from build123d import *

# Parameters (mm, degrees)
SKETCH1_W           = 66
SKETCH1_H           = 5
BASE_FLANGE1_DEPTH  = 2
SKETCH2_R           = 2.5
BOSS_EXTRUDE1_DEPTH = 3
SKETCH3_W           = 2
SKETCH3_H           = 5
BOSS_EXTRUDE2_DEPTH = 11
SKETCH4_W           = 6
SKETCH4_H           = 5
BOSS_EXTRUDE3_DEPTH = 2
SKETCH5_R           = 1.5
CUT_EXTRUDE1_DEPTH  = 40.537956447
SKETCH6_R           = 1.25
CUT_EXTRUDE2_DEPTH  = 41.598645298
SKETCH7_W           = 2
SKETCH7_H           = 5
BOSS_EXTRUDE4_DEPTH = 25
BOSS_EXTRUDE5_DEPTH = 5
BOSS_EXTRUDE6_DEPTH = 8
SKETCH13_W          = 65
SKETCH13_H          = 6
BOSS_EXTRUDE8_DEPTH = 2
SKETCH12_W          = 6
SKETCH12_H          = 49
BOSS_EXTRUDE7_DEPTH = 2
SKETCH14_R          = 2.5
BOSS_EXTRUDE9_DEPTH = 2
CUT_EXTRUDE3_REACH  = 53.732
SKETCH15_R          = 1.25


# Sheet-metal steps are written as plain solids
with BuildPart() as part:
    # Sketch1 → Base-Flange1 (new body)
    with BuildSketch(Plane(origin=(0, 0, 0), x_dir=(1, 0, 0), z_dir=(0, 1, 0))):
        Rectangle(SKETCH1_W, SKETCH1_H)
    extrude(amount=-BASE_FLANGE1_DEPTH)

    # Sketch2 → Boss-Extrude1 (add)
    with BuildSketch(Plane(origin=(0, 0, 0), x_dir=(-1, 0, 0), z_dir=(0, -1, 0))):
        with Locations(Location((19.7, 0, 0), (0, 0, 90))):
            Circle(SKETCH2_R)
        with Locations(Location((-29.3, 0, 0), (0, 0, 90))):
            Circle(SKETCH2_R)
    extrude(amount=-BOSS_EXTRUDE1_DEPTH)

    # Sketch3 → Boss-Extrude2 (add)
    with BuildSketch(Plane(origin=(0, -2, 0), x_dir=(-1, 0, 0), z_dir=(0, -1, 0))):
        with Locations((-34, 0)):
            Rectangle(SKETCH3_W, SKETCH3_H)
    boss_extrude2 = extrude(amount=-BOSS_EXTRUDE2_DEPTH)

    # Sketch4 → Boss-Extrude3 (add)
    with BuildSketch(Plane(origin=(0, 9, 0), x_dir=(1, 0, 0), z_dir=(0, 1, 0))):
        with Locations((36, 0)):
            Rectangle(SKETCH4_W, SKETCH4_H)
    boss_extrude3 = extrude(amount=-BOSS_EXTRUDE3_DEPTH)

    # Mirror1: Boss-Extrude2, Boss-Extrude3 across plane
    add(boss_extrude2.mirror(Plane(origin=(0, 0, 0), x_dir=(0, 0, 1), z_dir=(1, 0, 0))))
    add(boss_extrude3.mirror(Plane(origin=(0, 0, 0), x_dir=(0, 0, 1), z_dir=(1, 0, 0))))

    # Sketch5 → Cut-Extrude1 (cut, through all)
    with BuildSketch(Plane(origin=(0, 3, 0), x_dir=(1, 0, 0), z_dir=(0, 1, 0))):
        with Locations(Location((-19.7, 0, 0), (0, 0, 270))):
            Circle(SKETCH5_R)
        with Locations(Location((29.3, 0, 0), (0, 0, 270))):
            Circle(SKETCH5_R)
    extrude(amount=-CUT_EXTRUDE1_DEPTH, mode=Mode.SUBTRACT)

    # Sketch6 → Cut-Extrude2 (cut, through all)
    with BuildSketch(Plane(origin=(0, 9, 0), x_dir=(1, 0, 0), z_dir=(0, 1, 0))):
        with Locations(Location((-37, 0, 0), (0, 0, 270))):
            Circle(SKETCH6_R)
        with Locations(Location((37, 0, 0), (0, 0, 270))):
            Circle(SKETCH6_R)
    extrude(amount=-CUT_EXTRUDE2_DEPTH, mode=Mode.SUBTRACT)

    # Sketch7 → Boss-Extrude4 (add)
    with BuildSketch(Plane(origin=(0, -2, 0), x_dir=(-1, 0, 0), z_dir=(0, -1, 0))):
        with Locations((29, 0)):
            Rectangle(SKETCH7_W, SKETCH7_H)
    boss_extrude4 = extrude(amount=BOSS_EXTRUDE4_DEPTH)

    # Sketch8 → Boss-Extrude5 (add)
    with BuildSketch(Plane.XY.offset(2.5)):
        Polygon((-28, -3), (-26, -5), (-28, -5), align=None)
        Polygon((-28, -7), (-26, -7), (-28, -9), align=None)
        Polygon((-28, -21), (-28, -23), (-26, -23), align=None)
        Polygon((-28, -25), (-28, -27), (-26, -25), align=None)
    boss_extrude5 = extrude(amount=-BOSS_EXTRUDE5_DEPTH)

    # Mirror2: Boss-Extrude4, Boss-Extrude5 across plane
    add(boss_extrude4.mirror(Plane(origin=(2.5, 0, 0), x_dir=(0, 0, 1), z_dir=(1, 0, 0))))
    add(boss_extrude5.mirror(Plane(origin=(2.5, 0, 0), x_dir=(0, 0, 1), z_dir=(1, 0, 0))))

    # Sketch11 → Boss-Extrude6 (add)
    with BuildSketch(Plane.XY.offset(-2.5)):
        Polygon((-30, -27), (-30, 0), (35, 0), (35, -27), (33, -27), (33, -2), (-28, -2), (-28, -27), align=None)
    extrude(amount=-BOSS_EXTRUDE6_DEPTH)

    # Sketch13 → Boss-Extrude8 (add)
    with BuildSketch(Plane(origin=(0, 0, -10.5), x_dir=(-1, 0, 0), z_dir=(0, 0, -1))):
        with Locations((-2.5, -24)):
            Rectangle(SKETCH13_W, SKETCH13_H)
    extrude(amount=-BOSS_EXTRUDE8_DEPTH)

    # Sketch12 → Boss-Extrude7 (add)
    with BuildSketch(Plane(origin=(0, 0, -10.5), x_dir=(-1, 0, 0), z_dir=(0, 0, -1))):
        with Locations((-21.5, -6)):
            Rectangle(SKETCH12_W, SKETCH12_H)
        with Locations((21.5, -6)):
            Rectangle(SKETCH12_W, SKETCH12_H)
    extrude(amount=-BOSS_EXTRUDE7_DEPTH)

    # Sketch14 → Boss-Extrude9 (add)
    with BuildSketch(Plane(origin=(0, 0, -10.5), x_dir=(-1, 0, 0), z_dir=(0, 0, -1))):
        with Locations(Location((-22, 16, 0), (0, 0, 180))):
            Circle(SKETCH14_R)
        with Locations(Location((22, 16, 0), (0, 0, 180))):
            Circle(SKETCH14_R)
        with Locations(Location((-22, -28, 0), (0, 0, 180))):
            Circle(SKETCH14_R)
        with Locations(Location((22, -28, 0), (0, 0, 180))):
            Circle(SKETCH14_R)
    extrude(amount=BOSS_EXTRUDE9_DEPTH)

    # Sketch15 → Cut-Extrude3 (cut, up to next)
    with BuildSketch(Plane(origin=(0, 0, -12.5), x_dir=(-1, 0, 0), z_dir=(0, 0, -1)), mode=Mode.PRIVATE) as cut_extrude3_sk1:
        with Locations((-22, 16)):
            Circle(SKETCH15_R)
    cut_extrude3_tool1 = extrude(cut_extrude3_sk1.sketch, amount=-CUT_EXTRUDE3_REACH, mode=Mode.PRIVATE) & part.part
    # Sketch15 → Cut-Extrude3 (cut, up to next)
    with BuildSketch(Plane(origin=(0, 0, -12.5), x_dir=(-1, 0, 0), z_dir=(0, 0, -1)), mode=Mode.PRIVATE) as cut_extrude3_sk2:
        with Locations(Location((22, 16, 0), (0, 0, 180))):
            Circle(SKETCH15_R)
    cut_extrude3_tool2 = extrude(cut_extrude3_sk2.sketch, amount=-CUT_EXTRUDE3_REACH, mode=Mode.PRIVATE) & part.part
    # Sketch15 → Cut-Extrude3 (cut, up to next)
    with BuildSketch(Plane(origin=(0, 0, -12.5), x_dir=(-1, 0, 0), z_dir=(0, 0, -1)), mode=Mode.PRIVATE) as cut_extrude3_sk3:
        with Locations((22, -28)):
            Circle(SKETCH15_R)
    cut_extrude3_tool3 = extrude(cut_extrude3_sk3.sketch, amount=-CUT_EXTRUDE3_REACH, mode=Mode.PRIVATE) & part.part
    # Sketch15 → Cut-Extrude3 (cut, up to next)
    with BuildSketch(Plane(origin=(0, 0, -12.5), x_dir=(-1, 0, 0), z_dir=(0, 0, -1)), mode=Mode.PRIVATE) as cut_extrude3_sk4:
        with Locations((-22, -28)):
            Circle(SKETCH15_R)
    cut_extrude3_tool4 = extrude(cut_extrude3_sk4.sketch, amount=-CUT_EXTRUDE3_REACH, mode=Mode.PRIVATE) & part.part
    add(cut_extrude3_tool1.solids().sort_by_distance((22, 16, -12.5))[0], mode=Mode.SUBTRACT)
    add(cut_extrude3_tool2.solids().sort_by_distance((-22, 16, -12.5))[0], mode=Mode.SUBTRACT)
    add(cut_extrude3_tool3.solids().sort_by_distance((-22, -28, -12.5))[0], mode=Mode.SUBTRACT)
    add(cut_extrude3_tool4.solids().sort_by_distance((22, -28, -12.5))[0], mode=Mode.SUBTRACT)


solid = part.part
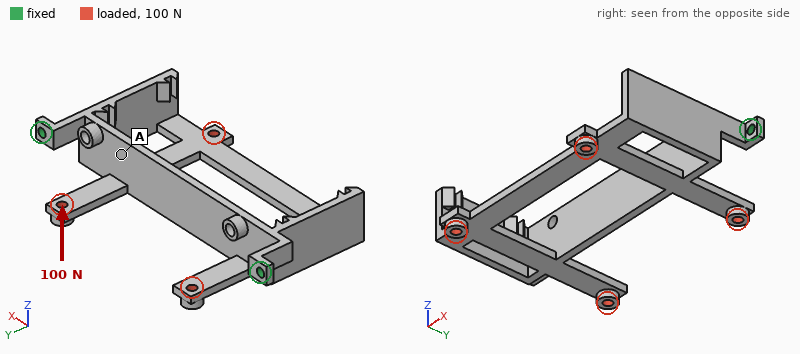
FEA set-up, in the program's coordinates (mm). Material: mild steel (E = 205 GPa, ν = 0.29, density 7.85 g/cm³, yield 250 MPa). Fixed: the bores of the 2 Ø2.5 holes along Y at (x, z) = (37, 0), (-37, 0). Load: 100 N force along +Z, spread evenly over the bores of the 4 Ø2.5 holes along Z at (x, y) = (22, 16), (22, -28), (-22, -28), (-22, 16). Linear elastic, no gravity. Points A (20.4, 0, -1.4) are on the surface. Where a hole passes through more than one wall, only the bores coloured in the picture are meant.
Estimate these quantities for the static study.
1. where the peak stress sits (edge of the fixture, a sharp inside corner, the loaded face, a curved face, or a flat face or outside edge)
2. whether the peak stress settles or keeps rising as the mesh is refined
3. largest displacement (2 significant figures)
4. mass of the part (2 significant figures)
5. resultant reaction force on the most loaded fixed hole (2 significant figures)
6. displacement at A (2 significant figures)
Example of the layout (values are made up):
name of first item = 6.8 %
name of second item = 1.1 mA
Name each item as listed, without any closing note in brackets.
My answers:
where the peak stress sits = edge of the fixture
whether the peak stress settles or keeps rising as the mesh is refined = keeps rising
largest displacement = 0.12 mm
mass of the part = 41 g
resultant reaction force on the most loaded fixed hole = 51 N
displacement at A = 0.019 mm
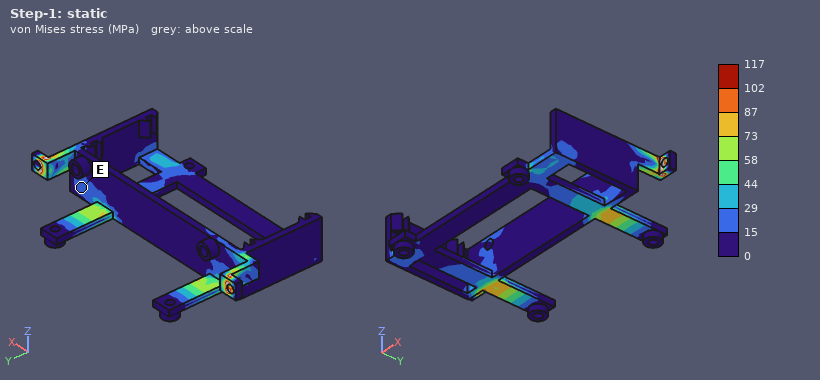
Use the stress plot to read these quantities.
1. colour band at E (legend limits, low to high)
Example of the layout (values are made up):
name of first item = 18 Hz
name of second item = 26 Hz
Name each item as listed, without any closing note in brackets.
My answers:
colour band at E = 15 to 29 MPa
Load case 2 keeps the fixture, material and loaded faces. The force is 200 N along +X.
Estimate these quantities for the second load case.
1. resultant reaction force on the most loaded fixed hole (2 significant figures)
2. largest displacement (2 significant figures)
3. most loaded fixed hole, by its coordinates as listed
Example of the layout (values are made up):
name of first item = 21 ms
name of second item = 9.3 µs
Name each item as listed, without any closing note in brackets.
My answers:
resultant reaction force on the most loaded fixed hole = 120 N
largest displacement = 43 µm
most loaded fixed hole, by its coordinates as listed = (37, 0)
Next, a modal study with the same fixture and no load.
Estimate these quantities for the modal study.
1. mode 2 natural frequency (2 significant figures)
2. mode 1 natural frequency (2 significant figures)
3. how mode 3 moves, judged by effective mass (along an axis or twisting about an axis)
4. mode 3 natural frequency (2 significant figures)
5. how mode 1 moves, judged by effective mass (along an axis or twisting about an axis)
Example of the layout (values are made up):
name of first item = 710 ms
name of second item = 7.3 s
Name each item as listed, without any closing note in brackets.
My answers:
mode 2 natural frequency = 1400 Hz
mode 1 natural frequency = 820 Hz
how mode 3 moves, judged by effective mass = along X
mode 3 natural frequency = 2100 Hz
how mode 1 moves, judged by effective mass = along Z
